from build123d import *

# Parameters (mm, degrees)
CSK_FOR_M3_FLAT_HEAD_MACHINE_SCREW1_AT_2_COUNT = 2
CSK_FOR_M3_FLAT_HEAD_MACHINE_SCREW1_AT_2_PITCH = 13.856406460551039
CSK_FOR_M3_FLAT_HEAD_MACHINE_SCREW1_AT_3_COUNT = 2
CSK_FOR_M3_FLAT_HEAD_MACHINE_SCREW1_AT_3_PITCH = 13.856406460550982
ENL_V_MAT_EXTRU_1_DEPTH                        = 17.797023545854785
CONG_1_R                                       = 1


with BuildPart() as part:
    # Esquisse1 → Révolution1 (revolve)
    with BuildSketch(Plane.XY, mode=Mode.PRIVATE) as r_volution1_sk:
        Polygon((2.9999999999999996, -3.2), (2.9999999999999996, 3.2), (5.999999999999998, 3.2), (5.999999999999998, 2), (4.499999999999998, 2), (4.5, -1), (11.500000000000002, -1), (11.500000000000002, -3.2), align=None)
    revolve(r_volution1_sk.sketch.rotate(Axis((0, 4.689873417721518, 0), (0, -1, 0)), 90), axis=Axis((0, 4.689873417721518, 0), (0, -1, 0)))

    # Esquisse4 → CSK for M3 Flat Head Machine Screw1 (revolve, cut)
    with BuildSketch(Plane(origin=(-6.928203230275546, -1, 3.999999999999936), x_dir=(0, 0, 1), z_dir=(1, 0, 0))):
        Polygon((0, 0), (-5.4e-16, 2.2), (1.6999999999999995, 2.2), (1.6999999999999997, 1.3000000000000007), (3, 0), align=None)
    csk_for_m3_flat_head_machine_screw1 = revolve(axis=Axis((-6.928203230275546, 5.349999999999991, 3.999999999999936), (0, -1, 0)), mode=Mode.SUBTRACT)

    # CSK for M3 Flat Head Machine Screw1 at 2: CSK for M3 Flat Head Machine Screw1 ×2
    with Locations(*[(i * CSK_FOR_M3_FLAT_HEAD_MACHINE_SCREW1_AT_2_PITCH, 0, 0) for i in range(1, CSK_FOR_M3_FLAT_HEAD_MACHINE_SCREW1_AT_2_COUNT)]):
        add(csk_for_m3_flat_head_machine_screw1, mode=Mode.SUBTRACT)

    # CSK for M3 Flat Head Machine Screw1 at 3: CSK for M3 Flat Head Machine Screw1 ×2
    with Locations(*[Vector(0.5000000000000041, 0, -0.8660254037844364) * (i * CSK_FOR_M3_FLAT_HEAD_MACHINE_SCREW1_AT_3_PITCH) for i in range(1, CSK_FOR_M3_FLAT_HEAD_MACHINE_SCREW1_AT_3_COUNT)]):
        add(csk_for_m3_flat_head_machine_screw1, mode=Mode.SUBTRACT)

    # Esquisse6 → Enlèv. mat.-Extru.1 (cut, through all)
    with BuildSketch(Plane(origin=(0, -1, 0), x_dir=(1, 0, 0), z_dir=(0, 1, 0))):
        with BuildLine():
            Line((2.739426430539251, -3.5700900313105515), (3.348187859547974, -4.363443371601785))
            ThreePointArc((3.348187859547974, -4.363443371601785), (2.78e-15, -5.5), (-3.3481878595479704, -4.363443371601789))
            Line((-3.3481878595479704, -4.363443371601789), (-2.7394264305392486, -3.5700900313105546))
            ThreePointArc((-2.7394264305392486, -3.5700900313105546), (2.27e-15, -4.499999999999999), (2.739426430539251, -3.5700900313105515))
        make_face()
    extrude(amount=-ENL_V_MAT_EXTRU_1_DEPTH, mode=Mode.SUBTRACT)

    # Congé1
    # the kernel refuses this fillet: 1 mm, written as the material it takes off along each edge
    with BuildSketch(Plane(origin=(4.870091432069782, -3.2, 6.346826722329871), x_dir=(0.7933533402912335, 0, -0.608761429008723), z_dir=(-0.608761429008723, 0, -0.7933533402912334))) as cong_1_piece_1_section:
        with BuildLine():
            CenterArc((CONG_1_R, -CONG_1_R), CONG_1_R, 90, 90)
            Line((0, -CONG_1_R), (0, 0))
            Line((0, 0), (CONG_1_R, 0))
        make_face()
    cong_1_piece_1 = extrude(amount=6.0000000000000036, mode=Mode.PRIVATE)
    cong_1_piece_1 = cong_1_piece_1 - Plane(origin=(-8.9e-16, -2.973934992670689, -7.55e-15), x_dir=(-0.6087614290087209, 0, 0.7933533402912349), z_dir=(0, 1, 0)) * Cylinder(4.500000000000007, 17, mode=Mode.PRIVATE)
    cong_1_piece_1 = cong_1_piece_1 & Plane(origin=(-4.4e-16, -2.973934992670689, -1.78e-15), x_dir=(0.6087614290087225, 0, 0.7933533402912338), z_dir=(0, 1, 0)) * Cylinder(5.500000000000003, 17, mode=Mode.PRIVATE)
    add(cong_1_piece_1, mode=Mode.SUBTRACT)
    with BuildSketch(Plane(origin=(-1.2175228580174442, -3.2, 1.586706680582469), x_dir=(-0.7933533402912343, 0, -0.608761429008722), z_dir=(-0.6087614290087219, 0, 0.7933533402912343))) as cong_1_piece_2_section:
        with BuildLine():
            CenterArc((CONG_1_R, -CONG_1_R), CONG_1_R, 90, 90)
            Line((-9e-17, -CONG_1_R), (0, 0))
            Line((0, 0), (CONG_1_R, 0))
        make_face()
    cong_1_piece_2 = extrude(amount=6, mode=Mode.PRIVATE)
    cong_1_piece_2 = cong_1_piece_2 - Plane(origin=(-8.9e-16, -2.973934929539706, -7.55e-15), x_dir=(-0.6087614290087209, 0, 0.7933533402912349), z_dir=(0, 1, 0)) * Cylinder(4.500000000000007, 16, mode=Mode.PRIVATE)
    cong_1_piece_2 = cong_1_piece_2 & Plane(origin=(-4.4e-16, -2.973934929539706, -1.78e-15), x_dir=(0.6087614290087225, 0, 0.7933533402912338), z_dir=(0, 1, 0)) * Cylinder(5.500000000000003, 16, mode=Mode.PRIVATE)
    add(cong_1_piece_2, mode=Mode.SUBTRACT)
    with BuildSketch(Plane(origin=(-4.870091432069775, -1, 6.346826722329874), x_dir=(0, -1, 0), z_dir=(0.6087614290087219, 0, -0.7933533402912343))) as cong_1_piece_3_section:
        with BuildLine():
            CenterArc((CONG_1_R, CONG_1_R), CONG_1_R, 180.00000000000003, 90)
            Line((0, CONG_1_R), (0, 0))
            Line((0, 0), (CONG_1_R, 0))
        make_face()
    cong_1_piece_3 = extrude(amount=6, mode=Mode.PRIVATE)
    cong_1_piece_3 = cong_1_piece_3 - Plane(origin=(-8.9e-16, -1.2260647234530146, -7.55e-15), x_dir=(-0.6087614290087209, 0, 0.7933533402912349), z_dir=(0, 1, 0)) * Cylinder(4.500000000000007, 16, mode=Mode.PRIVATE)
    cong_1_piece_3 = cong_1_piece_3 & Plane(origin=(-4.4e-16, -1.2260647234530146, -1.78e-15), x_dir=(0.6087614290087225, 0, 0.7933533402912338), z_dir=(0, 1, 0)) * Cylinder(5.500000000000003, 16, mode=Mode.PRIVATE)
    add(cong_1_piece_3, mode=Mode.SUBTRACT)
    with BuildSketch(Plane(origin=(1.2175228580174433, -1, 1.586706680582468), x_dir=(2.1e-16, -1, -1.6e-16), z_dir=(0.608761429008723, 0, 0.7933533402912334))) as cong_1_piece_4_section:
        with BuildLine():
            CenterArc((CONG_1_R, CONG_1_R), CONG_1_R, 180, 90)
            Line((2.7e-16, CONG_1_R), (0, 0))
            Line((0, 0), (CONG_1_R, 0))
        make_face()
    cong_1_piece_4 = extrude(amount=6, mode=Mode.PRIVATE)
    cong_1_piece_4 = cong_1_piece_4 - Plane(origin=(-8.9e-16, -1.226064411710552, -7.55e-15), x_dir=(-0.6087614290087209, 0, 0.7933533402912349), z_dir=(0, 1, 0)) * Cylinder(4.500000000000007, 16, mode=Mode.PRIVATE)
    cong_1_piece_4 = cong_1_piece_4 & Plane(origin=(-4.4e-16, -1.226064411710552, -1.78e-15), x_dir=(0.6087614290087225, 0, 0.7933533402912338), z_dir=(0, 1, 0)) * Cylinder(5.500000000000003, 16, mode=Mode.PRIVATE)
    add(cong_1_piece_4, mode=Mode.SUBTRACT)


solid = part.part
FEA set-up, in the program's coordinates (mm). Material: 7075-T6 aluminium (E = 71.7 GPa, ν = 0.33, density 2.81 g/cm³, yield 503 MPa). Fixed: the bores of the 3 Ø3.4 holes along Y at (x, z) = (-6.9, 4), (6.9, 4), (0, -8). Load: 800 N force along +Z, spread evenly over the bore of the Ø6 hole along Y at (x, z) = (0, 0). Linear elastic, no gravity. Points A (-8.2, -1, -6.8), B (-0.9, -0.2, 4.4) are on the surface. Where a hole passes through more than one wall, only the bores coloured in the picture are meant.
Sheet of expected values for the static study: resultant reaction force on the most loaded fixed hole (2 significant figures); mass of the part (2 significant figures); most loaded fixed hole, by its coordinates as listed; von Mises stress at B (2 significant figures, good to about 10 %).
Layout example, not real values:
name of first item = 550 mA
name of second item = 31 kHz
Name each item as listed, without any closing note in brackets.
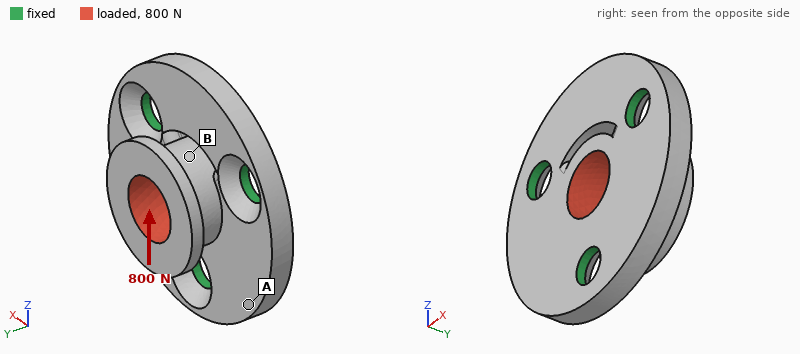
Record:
resultant reaction force on the most loaded fixed hole = 390 N
mass of the part = 2.7 g
most loaded fixed hole, by its coordinates as listed = (0, -8)
von Mises stress at B = 21 MPa
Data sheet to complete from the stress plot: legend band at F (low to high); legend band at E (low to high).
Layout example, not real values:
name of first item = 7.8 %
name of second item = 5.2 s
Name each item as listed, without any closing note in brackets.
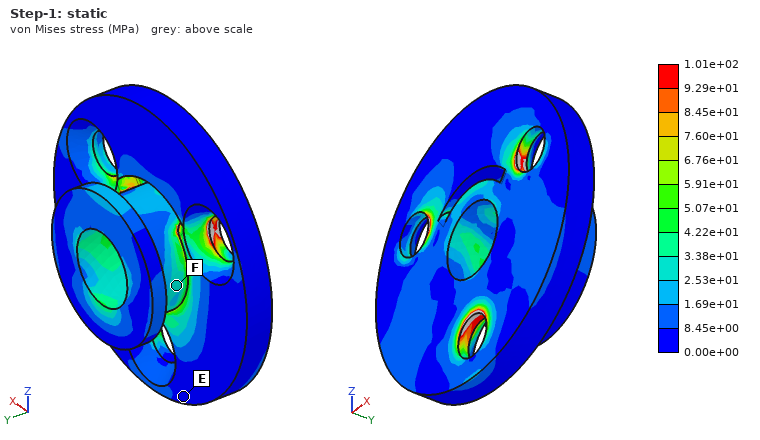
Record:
legend band at F = 2.53e+01 to 3.38e+01 MPa
legend band at E = 0.00e+00 to 8.45e+00 MPa
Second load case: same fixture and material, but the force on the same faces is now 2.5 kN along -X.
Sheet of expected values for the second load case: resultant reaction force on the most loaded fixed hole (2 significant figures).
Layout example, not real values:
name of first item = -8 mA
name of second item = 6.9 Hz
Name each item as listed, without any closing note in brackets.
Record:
resultant reaction force on the most loaded fixed hole = 1.0 kN
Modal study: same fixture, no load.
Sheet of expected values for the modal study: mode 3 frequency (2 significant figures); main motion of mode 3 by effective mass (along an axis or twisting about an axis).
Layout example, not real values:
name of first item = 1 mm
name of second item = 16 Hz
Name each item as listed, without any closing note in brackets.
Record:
mode 3 frequency = 30 kHz
main motion of mode 3 by effective mass = along Y
